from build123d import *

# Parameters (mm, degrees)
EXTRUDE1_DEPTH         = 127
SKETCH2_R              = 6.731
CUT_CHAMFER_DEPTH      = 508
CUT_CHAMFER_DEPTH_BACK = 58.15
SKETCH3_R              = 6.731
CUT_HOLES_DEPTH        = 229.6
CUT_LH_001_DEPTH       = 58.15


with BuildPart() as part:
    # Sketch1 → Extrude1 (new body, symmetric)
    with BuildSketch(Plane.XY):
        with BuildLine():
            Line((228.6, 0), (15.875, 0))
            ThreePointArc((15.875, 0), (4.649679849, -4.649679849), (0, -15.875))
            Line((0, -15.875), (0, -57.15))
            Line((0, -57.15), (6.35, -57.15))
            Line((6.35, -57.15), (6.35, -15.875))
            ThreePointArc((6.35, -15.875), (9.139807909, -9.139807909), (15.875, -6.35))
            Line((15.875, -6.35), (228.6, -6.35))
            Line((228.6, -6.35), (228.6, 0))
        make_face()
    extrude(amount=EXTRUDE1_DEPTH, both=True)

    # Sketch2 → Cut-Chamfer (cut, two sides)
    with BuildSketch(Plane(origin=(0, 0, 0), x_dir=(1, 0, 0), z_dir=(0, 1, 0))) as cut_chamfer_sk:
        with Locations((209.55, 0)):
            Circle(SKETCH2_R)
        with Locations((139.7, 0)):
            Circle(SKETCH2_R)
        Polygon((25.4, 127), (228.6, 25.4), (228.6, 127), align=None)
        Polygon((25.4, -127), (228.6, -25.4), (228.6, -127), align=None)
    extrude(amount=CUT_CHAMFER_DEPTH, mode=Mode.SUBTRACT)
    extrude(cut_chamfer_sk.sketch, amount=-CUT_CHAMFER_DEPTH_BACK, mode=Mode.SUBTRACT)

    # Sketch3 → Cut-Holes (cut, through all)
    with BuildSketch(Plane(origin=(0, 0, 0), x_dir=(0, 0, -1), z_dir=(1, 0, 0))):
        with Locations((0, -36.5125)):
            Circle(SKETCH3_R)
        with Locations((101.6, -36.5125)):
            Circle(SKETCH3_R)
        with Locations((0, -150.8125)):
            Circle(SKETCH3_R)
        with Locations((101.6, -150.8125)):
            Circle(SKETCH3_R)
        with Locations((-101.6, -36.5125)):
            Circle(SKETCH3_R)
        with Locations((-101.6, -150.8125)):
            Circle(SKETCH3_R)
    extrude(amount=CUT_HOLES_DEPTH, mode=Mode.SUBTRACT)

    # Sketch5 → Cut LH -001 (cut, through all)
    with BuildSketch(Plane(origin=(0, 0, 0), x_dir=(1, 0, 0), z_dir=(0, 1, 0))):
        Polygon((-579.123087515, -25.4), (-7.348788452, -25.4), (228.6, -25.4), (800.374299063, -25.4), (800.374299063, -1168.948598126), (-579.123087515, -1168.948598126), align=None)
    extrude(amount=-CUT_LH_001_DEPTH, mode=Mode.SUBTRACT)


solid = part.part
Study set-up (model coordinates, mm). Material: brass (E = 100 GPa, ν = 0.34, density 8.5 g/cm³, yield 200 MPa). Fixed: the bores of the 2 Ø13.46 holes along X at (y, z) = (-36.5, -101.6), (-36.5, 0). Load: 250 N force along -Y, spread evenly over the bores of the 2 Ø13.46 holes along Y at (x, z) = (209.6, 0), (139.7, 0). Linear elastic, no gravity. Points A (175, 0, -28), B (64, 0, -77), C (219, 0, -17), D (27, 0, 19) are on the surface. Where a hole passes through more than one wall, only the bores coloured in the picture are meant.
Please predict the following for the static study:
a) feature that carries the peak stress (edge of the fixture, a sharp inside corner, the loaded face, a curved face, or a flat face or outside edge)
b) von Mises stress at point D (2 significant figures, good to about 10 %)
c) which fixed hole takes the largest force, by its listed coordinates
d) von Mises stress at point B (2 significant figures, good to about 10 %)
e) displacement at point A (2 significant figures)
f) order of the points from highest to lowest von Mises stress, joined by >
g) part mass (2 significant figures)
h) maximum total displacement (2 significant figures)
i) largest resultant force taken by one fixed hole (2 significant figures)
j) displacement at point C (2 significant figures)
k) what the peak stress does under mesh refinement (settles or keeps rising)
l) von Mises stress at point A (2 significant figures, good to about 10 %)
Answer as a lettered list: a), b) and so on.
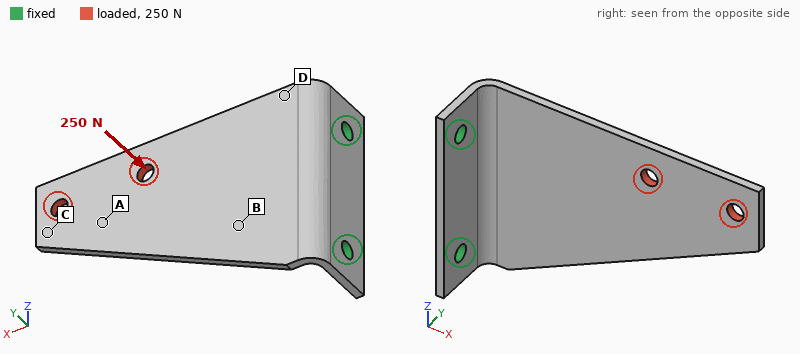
a) edge of the fixture
b) 43 MPa
c) (-36.5, 0)
d) 32 MPa
e) 2.1 mm
f) D > B > A > C
g) 1.7 kg
h) 3.3 mm
i) 260 N
j) 2.9 mm
k) keeps rising
l) 12 MPa
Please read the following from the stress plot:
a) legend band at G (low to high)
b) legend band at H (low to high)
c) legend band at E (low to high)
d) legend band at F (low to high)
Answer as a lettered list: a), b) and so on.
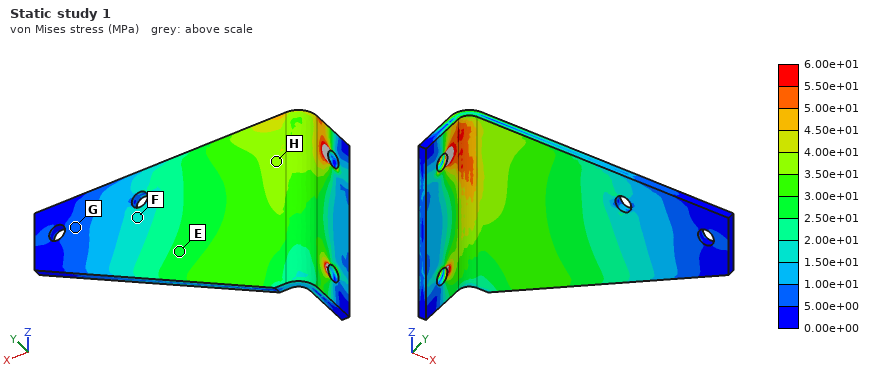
a) 5.00e+00 to 1.00e+01 MPa
b) 3.50e+01 to 4.00e+01 MPa
c) 2.50e+01 to 3.00e+01 MPa
d) 1.50e+01 to 2.00e+01 MPa
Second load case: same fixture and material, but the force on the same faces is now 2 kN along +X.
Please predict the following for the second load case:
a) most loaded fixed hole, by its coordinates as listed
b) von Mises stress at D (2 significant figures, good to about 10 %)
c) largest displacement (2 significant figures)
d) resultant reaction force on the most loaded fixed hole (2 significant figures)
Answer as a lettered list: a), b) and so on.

a) (-36.5, 0)
b) 14 MPa
c) 0.93 mm
d) 2.0 kN
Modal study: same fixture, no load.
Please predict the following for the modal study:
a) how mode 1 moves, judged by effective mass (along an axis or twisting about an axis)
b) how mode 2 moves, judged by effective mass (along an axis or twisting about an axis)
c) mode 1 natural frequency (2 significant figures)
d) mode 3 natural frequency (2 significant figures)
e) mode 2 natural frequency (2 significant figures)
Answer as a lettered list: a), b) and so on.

a) along Y
b) along Z
c) 79 Hz
d) 380 Hz
e) 350 Hz
